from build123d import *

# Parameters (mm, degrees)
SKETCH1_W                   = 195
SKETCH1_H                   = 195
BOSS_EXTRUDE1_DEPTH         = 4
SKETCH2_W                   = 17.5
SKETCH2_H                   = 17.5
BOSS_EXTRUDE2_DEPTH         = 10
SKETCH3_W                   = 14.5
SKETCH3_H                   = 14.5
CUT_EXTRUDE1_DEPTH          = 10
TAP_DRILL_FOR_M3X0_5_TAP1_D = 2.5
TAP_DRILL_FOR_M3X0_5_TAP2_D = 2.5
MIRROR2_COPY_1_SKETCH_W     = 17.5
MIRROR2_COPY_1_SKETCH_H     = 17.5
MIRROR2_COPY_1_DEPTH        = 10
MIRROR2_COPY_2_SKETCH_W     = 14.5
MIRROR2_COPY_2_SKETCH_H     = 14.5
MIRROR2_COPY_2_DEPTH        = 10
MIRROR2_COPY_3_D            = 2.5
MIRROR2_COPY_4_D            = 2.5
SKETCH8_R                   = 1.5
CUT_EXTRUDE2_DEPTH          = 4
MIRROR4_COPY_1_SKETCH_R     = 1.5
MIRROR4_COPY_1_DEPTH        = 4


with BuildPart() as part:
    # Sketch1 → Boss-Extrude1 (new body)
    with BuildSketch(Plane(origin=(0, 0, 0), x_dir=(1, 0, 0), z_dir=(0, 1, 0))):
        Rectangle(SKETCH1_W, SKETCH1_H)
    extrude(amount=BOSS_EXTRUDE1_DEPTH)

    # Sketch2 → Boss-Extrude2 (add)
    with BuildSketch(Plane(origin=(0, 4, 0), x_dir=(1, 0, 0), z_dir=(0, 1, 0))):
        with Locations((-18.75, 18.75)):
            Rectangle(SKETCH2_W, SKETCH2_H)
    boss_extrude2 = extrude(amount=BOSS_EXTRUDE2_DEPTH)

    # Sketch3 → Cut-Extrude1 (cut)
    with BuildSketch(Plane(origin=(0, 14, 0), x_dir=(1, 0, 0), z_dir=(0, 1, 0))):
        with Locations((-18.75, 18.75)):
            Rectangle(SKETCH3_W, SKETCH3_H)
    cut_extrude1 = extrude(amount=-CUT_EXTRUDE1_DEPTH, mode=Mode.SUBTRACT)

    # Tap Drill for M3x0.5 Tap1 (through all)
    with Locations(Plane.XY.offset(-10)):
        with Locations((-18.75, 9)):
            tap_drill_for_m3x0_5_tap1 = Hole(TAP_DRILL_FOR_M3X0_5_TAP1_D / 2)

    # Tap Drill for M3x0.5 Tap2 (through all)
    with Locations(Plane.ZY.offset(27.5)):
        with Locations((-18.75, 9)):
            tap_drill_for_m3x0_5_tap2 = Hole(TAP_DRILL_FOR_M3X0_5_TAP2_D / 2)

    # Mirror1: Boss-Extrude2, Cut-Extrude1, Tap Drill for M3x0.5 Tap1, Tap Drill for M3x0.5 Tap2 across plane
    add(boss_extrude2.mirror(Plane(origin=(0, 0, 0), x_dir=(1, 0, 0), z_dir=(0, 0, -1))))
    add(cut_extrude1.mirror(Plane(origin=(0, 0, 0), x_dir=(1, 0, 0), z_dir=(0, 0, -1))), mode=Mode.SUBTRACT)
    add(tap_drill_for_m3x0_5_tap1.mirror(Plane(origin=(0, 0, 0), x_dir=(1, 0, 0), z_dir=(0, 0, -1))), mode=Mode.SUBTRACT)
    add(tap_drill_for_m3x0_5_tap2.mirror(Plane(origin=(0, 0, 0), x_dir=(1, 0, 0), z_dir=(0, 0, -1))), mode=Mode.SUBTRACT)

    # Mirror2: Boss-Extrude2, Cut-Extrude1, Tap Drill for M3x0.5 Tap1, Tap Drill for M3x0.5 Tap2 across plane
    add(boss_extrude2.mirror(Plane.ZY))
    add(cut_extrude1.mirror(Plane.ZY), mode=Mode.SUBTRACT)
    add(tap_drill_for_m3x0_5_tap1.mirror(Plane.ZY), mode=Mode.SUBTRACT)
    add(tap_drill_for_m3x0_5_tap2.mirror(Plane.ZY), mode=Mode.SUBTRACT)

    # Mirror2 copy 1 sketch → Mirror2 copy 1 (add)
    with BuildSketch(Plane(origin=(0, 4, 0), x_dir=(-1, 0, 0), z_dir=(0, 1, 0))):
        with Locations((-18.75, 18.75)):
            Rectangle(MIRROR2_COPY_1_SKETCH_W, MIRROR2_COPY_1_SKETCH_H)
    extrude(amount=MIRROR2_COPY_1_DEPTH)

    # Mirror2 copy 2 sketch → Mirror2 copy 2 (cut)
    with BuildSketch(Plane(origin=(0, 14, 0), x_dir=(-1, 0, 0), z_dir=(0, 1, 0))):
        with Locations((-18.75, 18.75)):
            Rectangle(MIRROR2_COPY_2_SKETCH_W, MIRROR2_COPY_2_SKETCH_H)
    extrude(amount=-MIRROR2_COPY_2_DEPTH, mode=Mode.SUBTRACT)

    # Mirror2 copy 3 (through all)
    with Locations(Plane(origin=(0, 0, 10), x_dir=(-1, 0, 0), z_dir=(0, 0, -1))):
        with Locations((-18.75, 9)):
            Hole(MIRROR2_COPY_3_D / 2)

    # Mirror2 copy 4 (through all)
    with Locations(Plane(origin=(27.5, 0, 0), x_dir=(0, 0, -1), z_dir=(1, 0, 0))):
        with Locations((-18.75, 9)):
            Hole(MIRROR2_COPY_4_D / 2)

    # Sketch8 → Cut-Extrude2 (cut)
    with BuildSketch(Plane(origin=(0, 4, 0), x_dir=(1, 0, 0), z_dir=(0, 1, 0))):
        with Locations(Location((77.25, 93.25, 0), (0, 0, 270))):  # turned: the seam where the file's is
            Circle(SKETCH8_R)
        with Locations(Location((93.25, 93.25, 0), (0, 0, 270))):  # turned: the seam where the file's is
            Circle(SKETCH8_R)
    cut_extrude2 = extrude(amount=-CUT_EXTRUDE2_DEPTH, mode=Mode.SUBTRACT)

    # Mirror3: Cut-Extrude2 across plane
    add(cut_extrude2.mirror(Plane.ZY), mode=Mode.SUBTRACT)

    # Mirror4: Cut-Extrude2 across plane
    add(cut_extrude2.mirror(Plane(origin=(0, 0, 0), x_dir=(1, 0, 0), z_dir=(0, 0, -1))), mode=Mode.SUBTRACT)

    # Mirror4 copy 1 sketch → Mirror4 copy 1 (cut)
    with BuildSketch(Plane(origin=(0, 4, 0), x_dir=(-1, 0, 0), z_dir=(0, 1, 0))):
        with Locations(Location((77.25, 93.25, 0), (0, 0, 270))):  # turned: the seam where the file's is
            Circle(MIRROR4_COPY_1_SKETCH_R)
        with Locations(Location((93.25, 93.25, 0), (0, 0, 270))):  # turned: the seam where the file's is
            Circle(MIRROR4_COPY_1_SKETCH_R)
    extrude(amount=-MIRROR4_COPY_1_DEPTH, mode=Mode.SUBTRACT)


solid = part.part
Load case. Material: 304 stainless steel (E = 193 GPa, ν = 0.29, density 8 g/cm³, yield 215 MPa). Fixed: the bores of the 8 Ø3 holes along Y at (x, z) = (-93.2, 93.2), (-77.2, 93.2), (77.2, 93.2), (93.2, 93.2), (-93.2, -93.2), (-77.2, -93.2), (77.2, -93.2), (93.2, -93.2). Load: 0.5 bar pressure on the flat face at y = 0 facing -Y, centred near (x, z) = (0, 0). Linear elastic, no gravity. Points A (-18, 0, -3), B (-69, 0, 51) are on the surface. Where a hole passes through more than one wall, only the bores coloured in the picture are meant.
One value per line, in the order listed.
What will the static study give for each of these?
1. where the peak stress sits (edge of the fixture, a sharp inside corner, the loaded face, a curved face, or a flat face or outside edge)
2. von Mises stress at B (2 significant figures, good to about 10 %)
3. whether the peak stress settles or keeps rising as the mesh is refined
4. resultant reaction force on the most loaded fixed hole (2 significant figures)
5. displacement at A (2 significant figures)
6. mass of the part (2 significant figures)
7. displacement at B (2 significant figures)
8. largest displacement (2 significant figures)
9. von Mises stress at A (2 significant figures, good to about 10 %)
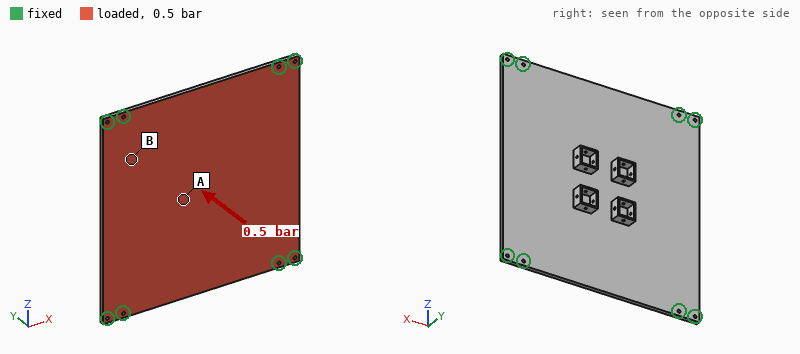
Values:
edge of the fixture
16 MPa
keeps rising
620 N
0.35 mm
1.2 kg
0.16 mm
0.36 mm
36 MPa
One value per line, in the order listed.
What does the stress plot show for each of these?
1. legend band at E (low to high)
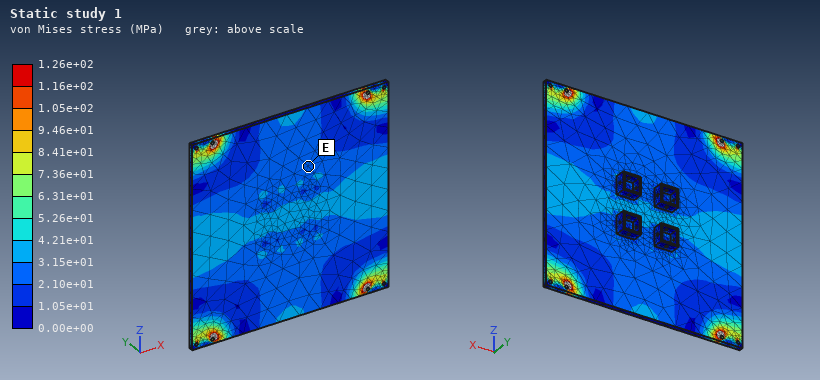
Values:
2.10e+01 to 3.15e+01 MPa
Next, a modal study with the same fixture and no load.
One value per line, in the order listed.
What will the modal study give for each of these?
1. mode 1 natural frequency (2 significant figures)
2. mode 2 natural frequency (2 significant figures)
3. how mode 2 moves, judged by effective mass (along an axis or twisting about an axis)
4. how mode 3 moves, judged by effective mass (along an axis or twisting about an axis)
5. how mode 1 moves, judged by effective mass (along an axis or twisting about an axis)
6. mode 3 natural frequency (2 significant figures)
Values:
390 Hz
640 Hz
twisting about Z
twisting about X
along Y
800 Hz
